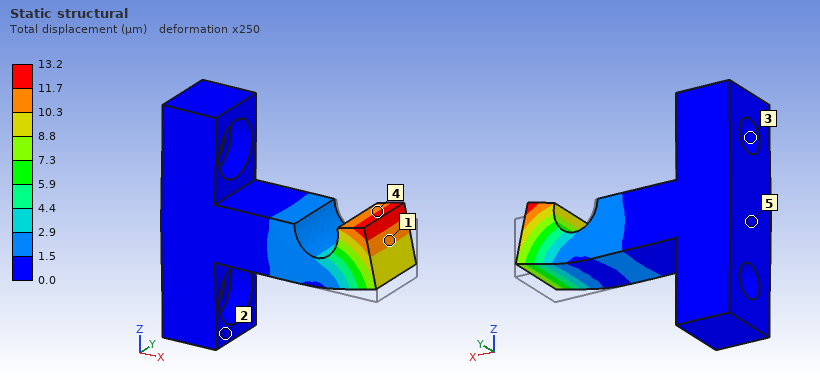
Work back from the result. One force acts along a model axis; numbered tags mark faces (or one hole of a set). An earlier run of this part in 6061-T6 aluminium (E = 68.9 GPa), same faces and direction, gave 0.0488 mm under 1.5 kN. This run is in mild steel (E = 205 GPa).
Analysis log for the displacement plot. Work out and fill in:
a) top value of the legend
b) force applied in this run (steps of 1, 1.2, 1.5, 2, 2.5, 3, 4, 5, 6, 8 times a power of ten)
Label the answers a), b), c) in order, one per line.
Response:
a) 13.2 µm
b) 1.2 kN
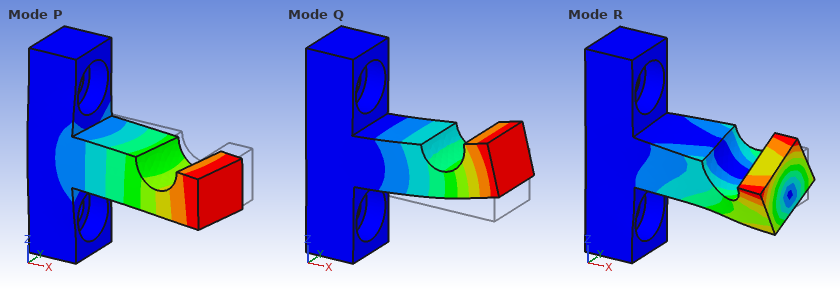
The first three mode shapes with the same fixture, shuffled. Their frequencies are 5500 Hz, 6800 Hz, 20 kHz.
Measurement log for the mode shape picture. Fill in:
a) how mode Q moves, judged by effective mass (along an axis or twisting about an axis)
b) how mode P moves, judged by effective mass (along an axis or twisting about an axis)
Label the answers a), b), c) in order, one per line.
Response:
a) along Z
b) along Y
